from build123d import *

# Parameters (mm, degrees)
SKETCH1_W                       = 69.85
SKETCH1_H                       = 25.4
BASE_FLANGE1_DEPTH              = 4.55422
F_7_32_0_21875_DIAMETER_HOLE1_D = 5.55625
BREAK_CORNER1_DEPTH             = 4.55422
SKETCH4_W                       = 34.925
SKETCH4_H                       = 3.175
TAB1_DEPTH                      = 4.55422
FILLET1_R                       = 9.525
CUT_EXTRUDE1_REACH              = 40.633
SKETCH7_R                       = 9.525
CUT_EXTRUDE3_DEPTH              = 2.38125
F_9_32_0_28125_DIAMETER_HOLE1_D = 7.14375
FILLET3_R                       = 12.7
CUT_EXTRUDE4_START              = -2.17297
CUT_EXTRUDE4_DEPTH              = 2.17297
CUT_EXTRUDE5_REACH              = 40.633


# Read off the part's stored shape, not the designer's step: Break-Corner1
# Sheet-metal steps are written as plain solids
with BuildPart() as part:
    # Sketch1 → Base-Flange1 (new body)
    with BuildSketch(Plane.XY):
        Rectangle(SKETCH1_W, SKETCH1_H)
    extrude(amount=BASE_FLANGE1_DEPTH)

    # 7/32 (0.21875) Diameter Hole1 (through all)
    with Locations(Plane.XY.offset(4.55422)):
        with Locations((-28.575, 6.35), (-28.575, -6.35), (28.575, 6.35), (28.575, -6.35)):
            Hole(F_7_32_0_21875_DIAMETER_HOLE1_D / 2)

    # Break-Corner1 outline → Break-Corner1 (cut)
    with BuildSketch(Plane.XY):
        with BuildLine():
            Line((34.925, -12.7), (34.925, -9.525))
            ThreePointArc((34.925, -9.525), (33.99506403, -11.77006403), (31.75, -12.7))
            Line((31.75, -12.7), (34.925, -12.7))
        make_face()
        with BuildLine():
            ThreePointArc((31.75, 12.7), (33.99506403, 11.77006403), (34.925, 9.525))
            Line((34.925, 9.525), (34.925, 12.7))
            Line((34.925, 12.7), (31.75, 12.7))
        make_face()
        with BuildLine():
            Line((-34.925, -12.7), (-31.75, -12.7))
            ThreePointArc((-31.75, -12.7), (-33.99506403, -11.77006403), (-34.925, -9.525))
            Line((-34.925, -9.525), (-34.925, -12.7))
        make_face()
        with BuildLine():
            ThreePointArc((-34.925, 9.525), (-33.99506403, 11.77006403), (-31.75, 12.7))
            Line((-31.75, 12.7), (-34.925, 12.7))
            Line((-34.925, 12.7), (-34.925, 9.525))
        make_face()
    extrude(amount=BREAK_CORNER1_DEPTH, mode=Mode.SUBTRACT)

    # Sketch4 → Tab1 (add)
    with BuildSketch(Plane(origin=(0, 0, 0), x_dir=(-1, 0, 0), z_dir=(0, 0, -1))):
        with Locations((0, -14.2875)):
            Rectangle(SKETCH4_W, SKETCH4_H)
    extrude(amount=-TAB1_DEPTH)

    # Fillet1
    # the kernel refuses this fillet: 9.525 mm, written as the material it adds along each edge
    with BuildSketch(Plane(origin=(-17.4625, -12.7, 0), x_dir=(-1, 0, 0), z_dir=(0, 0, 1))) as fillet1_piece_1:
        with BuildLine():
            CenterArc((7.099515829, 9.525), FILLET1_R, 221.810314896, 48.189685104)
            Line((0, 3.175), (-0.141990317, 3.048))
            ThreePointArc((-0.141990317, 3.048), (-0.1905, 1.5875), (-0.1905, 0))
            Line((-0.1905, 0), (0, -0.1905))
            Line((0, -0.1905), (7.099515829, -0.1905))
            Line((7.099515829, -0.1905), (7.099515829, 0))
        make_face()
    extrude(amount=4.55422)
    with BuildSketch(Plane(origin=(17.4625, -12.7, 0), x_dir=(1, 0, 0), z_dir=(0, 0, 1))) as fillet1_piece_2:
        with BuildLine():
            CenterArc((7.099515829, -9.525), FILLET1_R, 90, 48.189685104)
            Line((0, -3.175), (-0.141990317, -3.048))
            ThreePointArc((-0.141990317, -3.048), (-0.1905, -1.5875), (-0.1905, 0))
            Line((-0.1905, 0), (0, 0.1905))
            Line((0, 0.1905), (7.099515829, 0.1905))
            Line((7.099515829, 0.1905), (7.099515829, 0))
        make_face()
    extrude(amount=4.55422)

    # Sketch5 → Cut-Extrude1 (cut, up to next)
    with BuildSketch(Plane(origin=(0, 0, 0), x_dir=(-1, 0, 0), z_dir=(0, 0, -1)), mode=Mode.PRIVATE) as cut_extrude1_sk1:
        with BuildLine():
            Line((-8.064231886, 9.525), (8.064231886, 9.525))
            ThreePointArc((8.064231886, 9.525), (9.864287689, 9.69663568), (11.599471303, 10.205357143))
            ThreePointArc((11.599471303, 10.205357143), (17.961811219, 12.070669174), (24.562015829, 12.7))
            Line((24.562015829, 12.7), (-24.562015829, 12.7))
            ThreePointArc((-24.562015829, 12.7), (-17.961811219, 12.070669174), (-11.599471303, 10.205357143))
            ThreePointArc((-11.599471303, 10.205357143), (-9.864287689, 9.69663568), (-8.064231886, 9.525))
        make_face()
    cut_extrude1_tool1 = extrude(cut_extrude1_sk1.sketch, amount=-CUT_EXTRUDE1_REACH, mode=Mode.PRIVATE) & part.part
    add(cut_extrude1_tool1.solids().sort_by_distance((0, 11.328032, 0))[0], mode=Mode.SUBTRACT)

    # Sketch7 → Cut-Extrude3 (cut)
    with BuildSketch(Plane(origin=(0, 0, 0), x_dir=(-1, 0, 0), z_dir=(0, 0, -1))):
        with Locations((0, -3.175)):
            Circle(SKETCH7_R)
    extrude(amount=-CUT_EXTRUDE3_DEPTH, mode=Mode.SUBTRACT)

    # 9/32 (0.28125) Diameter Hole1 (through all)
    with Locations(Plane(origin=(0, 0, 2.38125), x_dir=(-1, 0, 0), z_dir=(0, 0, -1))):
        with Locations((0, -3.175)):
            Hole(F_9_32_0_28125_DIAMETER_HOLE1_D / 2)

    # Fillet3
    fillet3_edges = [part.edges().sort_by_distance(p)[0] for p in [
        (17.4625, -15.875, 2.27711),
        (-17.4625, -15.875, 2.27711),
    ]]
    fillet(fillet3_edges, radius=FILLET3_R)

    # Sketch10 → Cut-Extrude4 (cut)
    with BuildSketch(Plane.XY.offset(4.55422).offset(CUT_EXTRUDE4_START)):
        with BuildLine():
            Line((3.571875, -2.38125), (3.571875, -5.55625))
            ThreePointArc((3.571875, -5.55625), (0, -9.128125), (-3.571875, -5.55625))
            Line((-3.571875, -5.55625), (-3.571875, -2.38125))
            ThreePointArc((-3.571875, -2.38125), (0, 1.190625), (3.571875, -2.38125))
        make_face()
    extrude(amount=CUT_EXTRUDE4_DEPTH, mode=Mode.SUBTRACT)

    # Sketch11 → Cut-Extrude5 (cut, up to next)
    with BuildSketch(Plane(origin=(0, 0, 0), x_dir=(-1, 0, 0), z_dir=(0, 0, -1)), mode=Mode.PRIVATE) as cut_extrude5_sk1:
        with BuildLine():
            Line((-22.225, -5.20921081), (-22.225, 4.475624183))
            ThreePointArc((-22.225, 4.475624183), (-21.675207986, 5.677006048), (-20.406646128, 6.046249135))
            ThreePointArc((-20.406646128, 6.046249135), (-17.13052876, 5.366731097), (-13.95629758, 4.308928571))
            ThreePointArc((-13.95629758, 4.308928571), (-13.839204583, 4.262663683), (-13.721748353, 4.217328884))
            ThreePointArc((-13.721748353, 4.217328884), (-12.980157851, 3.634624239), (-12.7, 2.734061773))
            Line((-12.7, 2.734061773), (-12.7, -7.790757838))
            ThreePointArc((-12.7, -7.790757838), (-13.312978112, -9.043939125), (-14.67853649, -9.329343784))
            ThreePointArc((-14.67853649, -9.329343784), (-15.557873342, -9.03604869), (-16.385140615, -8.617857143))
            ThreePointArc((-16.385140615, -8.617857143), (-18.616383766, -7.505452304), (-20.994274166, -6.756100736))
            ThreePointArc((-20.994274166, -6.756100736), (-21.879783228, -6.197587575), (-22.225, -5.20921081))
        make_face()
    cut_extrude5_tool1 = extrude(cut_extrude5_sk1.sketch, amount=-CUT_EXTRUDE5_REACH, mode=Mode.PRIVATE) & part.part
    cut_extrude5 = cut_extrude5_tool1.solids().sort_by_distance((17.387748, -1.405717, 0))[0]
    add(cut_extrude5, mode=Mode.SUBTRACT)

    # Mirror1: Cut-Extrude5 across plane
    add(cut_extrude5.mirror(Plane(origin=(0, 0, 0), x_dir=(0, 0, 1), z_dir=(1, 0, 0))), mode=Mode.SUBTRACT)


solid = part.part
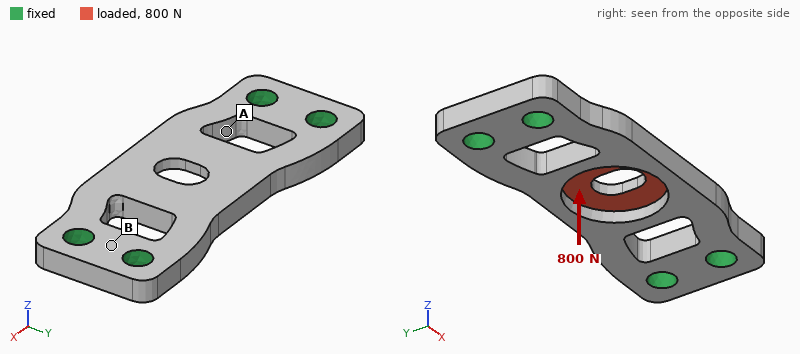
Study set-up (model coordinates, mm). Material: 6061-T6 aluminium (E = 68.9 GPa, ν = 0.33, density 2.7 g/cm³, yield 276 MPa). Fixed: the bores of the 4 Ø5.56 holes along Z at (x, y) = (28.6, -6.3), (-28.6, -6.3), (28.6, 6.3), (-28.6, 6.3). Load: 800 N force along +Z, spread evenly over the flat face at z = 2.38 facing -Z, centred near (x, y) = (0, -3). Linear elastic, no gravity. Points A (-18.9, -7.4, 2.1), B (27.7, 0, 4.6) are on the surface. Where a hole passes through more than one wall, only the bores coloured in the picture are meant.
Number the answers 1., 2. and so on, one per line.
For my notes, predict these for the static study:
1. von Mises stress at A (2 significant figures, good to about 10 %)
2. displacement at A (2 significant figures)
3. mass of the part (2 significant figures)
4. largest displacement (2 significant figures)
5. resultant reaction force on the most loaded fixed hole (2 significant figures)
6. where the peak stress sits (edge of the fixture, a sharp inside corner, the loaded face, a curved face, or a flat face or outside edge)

1. 45 MPa
2. 0.018 mm
3. 16 g
4. 0.10 mm
5. 260 N
6. a curved face
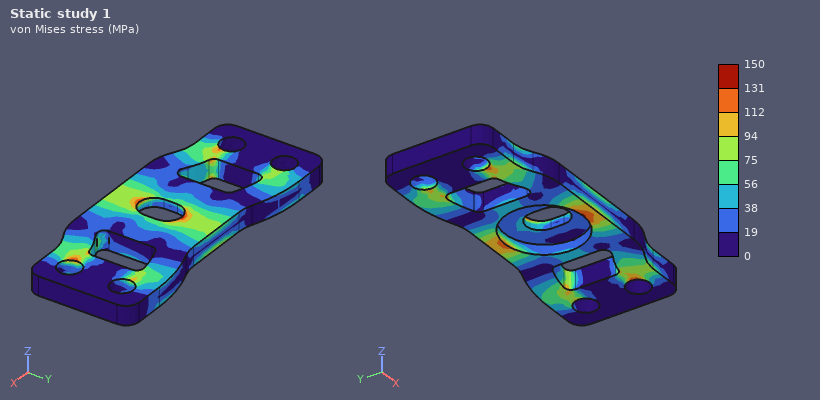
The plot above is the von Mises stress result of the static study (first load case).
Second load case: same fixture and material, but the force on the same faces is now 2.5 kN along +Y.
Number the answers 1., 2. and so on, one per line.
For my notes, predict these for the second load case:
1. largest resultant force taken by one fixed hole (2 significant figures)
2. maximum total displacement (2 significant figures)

1. 1.0 kN
2. 52 µm
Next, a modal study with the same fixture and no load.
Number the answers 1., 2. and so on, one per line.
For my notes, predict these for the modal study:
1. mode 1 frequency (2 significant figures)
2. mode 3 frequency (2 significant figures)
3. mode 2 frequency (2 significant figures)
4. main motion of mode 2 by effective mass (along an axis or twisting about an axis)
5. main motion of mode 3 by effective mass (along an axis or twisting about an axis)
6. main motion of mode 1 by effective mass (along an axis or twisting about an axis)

1. 6900 Hz
2. 15 kHz
3. 10 kHz
4. twisting about X
5. along Y
6. along Z
